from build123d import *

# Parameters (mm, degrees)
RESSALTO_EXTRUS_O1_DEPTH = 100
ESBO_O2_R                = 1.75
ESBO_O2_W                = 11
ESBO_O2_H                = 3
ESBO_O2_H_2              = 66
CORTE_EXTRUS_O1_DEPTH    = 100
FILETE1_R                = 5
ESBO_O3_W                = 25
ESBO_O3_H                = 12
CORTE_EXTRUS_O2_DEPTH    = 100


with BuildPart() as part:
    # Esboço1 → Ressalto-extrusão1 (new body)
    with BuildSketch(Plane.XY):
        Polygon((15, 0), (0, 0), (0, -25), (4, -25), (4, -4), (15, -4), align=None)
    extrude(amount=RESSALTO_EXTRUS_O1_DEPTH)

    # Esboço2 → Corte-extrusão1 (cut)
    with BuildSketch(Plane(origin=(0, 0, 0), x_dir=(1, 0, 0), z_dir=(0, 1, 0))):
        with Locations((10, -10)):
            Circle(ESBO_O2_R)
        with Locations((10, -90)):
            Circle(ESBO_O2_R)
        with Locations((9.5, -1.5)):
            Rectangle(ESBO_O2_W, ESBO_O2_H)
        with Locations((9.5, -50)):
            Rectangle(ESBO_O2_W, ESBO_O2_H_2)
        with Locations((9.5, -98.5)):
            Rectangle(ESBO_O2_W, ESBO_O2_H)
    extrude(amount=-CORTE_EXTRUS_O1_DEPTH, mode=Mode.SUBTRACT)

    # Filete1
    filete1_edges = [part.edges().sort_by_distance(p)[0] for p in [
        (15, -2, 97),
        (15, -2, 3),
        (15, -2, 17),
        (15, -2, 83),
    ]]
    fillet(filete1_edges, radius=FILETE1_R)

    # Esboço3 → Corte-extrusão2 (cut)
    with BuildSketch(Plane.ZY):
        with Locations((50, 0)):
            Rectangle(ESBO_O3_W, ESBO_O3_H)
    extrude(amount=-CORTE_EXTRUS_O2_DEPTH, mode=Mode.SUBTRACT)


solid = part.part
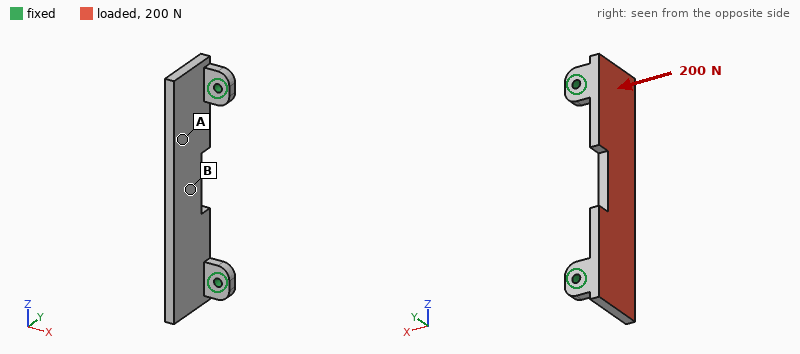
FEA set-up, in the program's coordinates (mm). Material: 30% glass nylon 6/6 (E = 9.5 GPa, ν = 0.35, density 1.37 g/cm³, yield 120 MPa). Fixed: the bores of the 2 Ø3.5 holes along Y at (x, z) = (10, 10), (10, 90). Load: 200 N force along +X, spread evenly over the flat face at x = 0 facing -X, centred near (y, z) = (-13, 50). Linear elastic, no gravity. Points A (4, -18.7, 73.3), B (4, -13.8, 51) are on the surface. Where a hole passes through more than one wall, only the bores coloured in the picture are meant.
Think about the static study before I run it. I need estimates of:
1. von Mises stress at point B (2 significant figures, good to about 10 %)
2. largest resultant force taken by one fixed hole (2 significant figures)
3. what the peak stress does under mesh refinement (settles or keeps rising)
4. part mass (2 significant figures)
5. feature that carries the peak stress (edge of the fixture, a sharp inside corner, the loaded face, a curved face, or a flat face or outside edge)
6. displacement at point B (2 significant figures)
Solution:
8.0 MPa
110 N
keeps rising
14 g
edge of the fixture
0.39 mm
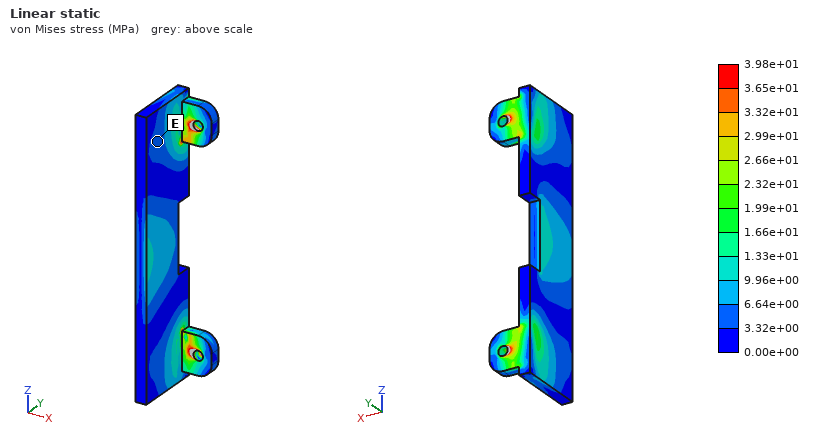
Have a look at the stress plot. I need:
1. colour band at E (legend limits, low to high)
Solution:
3.32e+00 to 6.64e+00 MPa
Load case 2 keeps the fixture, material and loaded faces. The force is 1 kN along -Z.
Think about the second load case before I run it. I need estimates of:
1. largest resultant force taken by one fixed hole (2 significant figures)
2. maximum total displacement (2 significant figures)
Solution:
520 N
0.14 mm
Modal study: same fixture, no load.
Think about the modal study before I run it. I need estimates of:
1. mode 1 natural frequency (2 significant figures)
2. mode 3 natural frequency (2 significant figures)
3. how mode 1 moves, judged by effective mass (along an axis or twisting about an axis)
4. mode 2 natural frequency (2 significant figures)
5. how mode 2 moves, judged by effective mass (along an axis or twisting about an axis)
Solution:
1000 Hz
2300 Hz
along X
2100 Hz
twisting about Y
